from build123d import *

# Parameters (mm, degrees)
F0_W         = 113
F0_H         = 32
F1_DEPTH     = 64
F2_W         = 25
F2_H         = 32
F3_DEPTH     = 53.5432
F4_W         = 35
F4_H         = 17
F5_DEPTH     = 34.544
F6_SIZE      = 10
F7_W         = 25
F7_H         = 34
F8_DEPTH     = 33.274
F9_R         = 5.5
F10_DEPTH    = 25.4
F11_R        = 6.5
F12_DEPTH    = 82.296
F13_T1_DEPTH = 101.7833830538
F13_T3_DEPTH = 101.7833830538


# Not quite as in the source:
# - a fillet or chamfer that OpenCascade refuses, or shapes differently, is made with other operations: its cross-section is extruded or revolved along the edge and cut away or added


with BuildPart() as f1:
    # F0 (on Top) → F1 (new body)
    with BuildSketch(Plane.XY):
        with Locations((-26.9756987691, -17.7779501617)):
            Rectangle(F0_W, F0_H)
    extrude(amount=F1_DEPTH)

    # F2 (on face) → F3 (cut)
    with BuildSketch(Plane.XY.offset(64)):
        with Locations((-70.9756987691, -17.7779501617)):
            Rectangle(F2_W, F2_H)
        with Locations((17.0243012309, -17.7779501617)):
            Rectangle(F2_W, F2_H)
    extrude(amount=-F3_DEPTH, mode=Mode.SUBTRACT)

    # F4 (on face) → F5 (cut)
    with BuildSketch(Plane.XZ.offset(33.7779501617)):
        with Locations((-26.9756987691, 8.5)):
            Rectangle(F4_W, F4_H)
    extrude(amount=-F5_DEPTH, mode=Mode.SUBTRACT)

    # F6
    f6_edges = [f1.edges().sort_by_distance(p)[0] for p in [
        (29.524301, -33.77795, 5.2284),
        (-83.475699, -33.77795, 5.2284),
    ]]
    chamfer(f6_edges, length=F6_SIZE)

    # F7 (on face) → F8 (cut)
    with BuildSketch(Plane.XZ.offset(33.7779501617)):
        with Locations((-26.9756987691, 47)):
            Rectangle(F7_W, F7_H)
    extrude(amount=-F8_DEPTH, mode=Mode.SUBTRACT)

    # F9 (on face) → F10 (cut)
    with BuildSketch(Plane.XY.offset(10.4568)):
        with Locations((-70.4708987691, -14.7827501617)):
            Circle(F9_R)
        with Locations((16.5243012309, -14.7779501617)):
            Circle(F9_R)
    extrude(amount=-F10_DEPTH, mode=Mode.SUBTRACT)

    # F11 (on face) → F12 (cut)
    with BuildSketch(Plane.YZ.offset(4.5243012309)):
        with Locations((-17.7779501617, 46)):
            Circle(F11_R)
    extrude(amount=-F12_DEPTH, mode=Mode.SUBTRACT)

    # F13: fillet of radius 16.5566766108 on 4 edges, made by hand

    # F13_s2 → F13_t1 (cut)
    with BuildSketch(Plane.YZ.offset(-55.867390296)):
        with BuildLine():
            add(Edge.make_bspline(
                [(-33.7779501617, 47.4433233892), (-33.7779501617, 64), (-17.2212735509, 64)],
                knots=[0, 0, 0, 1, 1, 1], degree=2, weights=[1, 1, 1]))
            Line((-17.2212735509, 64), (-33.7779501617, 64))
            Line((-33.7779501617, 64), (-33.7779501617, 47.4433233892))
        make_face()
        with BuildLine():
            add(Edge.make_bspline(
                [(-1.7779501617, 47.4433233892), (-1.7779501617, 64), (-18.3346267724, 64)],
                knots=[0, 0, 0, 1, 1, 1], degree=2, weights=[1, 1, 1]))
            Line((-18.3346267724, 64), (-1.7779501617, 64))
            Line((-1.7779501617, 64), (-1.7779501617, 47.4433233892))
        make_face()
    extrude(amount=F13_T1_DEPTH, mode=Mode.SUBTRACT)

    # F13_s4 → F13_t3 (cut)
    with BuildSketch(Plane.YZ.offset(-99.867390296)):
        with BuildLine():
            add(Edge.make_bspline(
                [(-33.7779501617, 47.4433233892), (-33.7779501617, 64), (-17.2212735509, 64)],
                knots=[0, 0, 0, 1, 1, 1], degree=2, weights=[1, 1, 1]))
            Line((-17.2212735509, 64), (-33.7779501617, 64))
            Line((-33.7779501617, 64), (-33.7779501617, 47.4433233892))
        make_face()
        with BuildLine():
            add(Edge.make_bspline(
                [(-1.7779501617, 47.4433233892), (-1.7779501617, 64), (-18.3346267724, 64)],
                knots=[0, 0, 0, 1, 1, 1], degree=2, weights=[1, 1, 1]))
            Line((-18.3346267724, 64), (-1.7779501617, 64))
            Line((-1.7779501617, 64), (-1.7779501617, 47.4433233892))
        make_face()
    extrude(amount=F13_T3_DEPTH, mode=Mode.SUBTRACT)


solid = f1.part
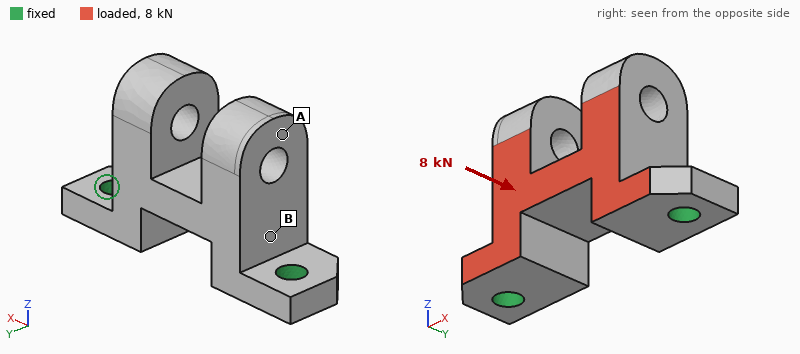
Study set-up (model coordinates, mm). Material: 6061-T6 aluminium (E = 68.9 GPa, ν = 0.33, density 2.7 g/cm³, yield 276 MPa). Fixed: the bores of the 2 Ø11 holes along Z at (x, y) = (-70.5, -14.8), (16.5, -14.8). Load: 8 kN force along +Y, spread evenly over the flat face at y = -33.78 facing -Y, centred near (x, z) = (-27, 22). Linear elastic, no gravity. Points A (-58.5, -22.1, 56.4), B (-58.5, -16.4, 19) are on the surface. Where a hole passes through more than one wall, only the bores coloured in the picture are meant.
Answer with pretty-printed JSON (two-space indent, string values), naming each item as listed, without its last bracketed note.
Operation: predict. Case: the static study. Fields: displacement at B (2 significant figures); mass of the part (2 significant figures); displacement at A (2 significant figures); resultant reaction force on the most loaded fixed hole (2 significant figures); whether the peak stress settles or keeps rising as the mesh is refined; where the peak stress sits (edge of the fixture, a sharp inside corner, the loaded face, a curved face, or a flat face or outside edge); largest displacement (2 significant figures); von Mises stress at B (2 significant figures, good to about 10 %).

{
  "displacement at B": "0.052 mm",
  "mass of the part": "240 g",
  "displacement at A": "0.17 mm",
  "resultant reaction force on the most loaded fixed hole": "4.0 kN",
  "whether the peak stress settles or keeps rising as the mesh is refined": "keeps rising",
  "where the peak stress sits": "edge of the fixture",
  "largest displacement": "0.19 mm",
  "von Mises stress at B": "27 MPa"
}
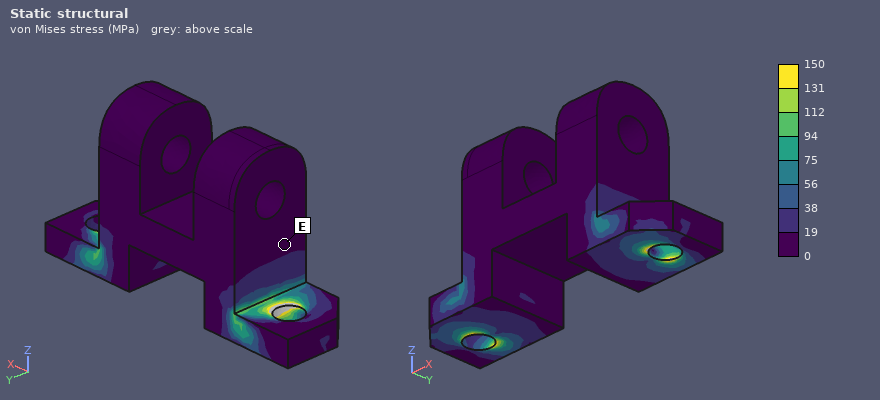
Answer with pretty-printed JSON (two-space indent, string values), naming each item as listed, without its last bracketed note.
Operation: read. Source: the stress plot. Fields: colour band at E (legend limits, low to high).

{
  "colour band at E": "0 to 19 MPa"
}
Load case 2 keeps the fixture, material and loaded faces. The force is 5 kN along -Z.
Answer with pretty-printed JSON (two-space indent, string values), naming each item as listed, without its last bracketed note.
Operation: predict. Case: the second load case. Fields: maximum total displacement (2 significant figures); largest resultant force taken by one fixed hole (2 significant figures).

{
  "maximum total displacement": "0.11 mm",
  "largest resultant force taken by one fixed hole": "2.9 kN"
}
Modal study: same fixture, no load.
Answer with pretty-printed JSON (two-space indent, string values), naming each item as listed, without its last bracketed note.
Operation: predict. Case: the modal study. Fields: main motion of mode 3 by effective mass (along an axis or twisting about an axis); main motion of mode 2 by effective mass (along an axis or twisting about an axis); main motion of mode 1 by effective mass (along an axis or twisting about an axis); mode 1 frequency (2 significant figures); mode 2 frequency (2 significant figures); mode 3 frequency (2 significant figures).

{
  "main motion of mode 3 by effective mass": "along X",
  "main motion of mode 2 by effective mass": "twisting about Z",
  "main motion of mode 1 by effective mass": "along Y",
  "mode 1 frequency": "2300 Hz",
  "mode 2 frequency": "4400 Hz",
  "mode 3 frequency": "5500 Hz"
}
